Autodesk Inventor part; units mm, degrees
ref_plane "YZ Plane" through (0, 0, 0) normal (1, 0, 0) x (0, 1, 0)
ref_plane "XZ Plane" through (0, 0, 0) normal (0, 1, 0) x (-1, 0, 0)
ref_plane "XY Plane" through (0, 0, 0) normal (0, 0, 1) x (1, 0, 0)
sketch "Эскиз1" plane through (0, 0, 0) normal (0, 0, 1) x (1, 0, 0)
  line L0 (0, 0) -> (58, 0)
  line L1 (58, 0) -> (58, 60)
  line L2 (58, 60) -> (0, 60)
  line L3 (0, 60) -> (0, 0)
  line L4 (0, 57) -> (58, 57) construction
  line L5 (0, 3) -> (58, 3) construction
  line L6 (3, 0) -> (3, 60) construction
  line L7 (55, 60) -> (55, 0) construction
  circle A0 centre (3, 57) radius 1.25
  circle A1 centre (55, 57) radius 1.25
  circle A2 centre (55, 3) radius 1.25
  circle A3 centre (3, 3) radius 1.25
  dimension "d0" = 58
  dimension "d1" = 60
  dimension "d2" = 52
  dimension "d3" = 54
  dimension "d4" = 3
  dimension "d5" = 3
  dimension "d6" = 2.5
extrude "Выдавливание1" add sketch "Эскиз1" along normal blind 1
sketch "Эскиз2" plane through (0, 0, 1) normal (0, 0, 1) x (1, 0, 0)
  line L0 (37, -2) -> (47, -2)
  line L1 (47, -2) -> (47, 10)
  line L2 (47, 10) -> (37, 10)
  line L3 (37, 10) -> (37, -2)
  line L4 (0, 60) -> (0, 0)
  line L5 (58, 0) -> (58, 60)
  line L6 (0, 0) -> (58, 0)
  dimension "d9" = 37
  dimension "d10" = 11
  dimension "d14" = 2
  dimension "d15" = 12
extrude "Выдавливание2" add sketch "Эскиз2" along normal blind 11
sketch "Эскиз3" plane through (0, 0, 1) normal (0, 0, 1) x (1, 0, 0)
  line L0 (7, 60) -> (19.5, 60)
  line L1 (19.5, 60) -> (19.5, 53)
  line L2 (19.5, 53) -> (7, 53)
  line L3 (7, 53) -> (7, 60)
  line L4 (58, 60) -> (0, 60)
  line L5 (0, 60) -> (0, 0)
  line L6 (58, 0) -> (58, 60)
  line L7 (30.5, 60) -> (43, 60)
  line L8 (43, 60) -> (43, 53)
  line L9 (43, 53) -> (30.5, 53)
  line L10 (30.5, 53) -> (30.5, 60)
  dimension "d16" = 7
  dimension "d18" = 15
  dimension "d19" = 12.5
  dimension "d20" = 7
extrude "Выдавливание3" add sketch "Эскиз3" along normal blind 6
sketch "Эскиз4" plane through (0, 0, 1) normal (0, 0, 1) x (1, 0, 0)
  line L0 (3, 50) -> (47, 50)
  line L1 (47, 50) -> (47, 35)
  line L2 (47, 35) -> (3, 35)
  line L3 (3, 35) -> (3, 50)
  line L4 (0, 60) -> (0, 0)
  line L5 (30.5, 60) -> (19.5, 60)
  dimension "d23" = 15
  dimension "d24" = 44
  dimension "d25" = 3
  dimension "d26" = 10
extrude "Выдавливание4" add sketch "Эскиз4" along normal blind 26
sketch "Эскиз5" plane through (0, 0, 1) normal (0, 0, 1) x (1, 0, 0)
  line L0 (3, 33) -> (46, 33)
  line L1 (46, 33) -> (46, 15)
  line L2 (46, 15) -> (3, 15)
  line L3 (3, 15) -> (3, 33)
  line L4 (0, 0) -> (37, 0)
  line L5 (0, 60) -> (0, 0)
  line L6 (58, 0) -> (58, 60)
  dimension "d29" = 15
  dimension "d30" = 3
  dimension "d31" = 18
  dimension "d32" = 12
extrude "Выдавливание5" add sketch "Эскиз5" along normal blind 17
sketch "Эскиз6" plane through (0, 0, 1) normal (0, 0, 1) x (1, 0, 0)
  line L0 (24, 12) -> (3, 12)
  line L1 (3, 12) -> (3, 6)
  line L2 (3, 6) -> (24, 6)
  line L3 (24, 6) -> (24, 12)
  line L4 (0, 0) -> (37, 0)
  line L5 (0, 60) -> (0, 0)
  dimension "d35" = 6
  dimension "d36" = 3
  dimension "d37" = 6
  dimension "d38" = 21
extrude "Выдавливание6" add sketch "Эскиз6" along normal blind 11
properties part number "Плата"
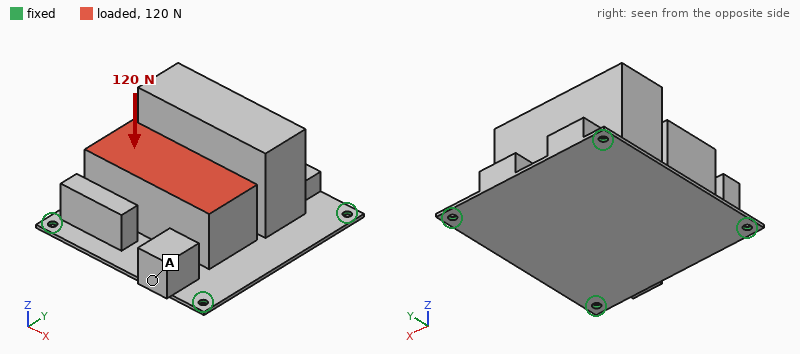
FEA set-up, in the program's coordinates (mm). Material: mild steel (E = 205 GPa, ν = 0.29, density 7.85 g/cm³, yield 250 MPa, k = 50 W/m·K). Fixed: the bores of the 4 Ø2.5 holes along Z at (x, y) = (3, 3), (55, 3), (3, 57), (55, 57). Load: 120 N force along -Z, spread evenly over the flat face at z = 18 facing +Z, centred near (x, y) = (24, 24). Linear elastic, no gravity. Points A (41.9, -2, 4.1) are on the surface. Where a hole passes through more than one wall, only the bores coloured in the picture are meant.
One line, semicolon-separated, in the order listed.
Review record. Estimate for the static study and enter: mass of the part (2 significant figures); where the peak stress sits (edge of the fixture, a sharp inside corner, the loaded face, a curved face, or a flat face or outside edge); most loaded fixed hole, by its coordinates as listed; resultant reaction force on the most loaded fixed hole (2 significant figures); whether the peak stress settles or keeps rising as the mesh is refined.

290 g; edge of the fixture; (3, 3); 62 N; keeps rising
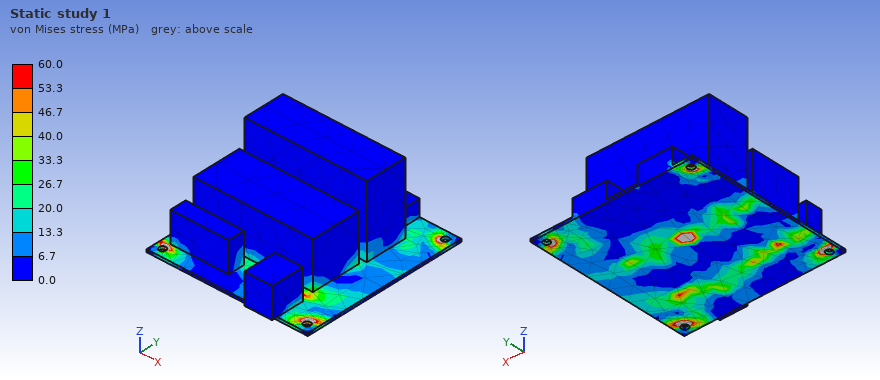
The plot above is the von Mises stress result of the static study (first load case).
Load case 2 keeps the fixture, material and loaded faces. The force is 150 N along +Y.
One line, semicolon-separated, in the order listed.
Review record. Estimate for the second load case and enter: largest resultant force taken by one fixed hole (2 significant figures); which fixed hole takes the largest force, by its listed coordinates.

78 N; (3, 57)
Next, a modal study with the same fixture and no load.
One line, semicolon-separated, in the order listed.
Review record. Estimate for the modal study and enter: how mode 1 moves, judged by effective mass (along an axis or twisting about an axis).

along Z
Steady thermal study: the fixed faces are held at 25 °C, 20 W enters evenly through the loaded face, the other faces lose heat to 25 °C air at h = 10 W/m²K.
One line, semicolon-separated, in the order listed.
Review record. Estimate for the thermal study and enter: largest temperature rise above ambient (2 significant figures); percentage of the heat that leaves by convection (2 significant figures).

75 K; 33 %
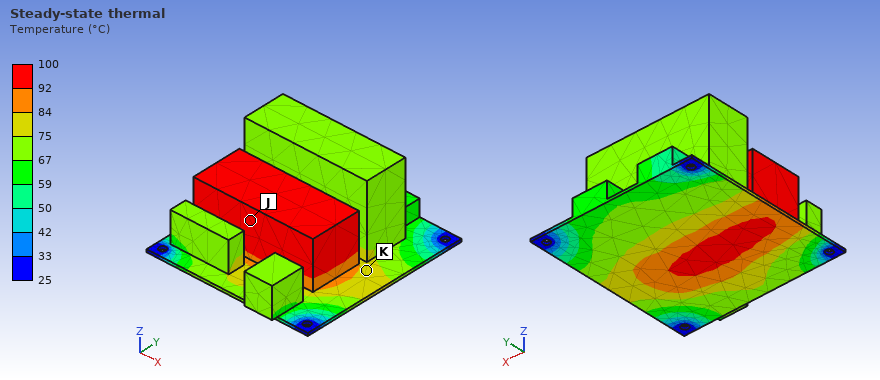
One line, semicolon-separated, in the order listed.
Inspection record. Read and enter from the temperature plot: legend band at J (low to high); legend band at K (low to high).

92 to 100 °C; 75 to 84 °C
